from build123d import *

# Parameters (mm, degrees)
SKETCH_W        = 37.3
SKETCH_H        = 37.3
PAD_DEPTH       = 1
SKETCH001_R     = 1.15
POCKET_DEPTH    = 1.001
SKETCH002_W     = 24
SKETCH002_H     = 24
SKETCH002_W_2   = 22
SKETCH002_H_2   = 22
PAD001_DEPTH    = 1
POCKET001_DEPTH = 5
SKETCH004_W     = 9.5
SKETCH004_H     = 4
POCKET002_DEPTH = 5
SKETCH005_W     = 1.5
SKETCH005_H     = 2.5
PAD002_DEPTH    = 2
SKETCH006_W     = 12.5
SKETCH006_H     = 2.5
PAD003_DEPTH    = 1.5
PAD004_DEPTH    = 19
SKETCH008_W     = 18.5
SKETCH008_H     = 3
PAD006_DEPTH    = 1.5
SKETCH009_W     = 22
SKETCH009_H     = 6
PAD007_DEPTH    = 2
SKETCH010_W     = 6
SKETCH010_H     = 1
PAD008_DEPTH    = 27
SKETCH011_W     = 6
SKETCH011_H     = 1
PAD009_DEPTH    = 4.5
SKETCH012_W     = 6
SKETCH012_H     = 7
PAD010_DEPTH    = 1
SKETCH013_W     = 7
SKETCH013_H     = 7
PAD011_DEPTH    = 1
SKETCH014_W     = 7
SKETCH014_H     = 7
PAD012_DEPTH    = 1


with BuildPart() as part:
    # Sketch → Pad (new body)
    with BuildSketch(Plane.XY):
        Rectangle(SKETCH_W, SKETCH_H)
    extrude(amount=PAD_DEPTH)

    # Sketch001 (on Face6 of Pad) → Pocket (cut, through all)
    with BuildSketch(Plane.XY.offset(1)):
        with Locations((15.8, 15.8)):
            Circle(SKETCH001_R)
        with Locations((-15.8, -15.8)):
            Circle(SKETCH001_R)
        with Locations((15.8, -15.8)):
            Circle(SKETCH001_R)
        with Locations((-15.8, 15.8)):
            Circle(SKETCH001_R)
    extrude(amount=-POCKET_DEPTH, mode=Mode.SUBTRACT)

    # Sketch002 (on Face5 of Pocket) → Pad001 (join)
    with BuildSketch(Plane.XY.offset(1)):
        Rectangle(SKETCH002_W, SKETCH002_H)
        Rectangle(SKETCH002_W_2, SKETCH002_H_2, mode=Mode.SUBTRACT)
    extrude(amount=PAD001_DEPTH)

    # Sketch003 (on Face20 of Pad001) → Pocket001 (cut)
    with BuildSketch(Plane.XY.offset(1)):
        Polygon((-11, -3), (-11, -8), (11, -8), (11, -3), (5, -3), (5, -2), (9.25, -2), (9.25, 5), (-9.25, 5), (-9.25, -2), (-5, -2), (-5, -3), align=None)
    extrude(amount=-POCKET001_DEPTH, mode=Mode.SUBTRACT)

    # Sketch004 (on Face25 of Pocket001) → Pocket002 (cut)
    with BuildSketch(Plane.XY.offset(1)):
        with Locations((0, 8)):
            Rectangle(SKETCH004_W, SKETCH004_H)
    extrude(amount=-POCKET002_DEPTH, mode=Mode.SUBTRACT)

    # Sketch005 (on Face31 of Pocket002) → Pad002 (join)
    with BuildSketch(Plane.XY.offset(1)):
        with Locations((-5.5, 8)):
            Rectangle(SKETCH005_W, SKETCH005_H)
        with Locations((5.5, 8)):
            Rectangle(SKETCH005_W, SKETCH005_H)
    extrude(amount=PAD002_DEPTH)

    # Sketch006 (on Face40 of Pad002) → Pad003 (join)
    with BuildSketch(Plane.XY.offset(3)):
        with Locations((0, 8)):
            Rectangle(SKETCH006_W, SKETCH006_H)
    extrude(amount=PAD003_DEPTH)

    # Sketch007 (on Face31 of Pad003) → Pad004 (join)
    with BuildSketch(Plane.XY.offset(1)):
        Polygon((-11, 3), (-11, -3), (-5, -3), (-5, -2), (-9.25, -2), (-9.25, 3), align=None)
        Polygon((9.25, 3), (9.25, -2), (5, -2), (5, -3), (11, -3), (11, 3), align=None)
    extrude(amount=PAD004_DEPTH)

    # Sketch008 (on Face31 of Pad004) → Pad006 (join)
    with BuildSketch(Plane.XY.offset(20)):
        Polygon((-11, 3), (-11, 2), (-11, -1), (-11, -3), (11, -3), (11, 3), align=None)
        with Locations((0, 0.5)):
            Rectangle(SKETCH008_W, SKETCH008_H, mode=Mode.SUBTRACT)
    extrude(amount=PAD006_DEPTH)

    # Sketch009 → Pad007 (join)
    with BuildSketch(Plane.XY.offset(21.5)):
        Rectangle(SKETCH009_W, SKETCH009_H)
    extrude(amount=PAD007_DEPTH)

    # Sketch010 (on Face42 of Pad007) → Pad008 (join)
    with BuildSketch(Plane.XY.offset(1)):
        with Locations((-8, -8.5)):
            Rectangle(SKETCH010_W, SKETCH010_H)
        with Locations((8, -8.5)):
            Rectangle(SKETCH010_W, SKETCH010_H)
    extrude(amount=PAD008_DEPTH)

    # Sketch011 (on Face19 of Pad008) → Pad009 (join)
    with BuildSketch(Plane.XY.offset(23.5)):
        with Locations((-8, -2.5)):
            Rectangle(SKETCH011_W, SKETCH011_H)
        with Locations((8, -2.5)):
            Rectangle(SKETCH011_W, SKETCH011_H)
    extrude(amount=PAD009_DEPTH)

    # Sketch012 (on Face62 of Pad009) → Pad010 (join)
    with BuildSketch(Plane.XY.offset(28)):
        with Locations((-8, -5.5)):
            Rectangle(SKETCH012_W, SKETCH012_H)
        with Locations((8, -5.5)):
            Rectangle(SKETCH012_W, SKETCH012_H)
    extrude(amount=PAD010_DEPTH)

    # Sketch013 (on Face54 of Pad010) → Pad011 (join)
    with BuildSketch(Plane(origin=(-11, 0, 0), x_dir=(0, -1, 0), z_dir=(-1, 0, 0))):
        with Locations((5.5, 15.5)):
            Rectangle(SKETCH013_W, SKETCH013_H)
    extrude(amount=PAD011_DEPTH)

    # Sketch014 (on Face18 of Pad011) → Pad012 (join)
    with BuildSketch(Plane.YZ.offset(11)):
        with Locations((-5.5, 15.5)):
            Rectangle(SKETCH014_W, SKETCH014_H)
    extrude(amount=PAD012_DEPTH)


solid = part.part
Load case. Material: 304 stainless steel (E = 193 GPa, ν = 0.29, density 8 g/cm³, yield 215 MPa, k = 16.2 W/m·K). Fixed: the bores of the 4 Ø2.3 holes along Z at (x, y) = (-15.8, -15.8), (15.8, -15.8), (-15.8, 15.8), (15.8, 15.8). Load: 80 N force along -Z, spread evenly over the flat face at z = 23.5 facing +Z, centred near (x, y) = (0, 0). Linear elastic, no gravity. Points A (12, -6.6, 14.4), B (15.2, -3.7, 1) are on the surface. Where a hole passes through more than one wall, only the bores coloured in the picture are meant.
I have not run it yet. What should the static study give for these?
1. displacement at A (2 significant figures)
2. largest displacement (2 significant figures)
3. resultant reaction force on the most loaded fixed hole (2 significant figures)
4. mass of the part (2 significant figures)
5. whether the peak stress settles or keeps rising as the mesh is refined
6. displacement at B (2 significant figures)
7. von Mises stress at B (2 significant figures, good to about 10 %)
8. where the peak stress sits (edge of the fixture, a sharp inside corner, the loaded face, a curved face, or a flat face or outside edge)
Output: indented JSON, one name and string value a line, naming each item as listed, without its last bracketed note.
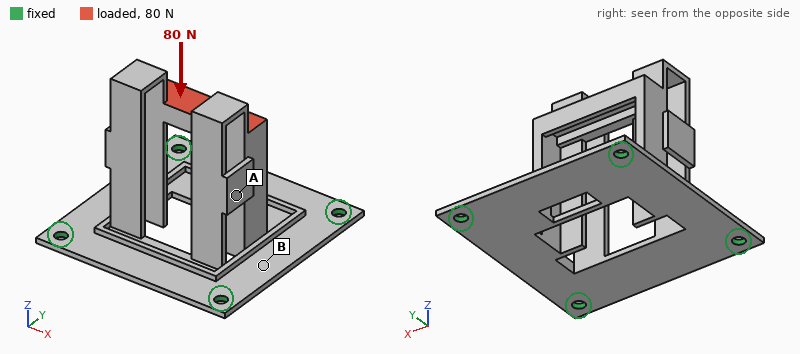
{
  "displacement at A": "15 µm",
  "largest displacement": "27 µm",
  "resultant reaction force on the most loaded fixed hole": "31 N",
  "mass of the part": "22 g",
  "whether the peak stress settles or keeps rising as the mesh is refined": "keeps rising",
  "displacement at B": "14 µm",
  "von Mises stress at B": "14 MPa",
  "where the peak stress sits": "a sharp inside corner"
}
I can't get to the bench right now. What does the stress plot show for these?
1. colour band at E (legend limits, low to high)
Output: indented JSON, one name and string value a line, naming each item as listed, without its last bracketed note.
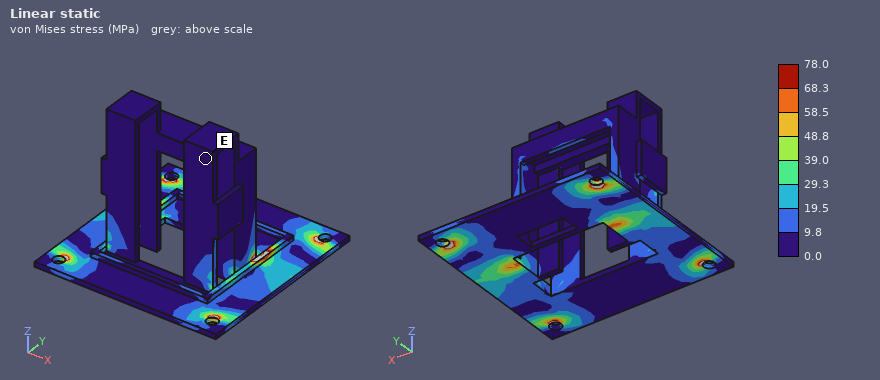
{
  "colour band at E": "0.0 to 9.8 MPa"
}
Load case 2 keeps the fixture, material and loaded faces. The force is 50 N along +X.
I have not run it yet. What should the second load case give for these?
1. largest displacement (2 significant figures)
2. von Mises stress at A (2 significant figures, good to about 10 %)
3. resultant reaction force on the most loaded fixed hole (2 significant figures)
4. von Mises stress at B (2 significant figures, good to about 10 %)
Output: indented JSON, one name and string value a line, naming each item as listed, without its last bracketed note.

{
  "largest displacement": "36 µm",
  "von Mises stress at A": "9.6 MPa",
  "resultant reaction force on the most loaded fixed hole": "35 N",
  "von Mises stress at B": "22 MPa"
}
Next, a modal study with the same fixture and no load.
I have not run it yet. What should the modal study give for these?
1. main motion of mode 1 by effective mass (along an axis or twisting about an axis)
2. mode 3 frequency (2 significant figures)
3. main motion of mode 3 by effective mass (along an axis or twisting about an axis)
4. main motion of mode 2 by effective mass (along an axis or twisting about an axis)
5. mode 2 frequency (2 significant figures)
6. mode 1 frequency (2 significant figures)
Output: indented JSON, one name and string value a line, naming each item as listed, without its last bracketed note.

{
  "main motion of mode 1 by effective mass": "along Y",
  "mode 3 frequency": "3200 Hz",
  "main motion of mode 3 by effective mass": "along Z",
  "main motion of mode 2 by effective mass": "along X",
  "mode 2 frequency": "2300 Hz",
  "mode 1 frequency": "2000 Hz"
}
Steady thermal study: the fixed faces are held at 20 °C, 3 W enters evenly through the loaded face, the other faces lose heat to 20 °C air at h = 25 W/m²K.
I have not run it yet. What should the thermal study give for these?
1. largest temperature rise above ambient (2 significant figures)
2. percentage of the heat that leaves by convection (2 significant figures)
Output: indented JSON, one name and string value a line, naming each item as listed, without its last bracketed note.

{
  "largest temperature rise above ambient": "74 K",
  "percentage of the heat that leaves by convection": "84 %"
}
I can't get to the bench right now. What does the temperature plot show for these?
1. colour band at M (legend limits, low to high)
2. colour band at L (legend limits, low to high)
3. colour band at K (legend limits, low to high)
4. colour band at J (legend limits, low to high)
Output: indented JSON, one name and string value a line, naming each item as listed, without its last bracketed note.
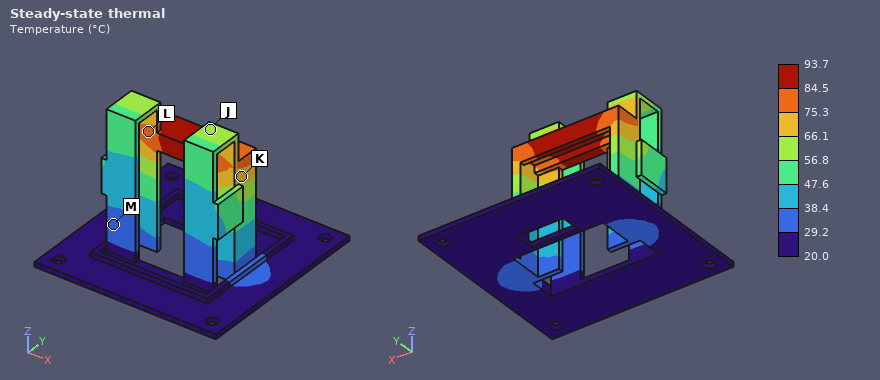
{
  "colour band at M": "29.2 to 38.4 °C",
  "colour band at L": "75.3 to 84.5 °C",
  "colour band at K": "66.1 to 75.3 °C",
  "colour band at J": "56.8 to 66.1 °C"
}
